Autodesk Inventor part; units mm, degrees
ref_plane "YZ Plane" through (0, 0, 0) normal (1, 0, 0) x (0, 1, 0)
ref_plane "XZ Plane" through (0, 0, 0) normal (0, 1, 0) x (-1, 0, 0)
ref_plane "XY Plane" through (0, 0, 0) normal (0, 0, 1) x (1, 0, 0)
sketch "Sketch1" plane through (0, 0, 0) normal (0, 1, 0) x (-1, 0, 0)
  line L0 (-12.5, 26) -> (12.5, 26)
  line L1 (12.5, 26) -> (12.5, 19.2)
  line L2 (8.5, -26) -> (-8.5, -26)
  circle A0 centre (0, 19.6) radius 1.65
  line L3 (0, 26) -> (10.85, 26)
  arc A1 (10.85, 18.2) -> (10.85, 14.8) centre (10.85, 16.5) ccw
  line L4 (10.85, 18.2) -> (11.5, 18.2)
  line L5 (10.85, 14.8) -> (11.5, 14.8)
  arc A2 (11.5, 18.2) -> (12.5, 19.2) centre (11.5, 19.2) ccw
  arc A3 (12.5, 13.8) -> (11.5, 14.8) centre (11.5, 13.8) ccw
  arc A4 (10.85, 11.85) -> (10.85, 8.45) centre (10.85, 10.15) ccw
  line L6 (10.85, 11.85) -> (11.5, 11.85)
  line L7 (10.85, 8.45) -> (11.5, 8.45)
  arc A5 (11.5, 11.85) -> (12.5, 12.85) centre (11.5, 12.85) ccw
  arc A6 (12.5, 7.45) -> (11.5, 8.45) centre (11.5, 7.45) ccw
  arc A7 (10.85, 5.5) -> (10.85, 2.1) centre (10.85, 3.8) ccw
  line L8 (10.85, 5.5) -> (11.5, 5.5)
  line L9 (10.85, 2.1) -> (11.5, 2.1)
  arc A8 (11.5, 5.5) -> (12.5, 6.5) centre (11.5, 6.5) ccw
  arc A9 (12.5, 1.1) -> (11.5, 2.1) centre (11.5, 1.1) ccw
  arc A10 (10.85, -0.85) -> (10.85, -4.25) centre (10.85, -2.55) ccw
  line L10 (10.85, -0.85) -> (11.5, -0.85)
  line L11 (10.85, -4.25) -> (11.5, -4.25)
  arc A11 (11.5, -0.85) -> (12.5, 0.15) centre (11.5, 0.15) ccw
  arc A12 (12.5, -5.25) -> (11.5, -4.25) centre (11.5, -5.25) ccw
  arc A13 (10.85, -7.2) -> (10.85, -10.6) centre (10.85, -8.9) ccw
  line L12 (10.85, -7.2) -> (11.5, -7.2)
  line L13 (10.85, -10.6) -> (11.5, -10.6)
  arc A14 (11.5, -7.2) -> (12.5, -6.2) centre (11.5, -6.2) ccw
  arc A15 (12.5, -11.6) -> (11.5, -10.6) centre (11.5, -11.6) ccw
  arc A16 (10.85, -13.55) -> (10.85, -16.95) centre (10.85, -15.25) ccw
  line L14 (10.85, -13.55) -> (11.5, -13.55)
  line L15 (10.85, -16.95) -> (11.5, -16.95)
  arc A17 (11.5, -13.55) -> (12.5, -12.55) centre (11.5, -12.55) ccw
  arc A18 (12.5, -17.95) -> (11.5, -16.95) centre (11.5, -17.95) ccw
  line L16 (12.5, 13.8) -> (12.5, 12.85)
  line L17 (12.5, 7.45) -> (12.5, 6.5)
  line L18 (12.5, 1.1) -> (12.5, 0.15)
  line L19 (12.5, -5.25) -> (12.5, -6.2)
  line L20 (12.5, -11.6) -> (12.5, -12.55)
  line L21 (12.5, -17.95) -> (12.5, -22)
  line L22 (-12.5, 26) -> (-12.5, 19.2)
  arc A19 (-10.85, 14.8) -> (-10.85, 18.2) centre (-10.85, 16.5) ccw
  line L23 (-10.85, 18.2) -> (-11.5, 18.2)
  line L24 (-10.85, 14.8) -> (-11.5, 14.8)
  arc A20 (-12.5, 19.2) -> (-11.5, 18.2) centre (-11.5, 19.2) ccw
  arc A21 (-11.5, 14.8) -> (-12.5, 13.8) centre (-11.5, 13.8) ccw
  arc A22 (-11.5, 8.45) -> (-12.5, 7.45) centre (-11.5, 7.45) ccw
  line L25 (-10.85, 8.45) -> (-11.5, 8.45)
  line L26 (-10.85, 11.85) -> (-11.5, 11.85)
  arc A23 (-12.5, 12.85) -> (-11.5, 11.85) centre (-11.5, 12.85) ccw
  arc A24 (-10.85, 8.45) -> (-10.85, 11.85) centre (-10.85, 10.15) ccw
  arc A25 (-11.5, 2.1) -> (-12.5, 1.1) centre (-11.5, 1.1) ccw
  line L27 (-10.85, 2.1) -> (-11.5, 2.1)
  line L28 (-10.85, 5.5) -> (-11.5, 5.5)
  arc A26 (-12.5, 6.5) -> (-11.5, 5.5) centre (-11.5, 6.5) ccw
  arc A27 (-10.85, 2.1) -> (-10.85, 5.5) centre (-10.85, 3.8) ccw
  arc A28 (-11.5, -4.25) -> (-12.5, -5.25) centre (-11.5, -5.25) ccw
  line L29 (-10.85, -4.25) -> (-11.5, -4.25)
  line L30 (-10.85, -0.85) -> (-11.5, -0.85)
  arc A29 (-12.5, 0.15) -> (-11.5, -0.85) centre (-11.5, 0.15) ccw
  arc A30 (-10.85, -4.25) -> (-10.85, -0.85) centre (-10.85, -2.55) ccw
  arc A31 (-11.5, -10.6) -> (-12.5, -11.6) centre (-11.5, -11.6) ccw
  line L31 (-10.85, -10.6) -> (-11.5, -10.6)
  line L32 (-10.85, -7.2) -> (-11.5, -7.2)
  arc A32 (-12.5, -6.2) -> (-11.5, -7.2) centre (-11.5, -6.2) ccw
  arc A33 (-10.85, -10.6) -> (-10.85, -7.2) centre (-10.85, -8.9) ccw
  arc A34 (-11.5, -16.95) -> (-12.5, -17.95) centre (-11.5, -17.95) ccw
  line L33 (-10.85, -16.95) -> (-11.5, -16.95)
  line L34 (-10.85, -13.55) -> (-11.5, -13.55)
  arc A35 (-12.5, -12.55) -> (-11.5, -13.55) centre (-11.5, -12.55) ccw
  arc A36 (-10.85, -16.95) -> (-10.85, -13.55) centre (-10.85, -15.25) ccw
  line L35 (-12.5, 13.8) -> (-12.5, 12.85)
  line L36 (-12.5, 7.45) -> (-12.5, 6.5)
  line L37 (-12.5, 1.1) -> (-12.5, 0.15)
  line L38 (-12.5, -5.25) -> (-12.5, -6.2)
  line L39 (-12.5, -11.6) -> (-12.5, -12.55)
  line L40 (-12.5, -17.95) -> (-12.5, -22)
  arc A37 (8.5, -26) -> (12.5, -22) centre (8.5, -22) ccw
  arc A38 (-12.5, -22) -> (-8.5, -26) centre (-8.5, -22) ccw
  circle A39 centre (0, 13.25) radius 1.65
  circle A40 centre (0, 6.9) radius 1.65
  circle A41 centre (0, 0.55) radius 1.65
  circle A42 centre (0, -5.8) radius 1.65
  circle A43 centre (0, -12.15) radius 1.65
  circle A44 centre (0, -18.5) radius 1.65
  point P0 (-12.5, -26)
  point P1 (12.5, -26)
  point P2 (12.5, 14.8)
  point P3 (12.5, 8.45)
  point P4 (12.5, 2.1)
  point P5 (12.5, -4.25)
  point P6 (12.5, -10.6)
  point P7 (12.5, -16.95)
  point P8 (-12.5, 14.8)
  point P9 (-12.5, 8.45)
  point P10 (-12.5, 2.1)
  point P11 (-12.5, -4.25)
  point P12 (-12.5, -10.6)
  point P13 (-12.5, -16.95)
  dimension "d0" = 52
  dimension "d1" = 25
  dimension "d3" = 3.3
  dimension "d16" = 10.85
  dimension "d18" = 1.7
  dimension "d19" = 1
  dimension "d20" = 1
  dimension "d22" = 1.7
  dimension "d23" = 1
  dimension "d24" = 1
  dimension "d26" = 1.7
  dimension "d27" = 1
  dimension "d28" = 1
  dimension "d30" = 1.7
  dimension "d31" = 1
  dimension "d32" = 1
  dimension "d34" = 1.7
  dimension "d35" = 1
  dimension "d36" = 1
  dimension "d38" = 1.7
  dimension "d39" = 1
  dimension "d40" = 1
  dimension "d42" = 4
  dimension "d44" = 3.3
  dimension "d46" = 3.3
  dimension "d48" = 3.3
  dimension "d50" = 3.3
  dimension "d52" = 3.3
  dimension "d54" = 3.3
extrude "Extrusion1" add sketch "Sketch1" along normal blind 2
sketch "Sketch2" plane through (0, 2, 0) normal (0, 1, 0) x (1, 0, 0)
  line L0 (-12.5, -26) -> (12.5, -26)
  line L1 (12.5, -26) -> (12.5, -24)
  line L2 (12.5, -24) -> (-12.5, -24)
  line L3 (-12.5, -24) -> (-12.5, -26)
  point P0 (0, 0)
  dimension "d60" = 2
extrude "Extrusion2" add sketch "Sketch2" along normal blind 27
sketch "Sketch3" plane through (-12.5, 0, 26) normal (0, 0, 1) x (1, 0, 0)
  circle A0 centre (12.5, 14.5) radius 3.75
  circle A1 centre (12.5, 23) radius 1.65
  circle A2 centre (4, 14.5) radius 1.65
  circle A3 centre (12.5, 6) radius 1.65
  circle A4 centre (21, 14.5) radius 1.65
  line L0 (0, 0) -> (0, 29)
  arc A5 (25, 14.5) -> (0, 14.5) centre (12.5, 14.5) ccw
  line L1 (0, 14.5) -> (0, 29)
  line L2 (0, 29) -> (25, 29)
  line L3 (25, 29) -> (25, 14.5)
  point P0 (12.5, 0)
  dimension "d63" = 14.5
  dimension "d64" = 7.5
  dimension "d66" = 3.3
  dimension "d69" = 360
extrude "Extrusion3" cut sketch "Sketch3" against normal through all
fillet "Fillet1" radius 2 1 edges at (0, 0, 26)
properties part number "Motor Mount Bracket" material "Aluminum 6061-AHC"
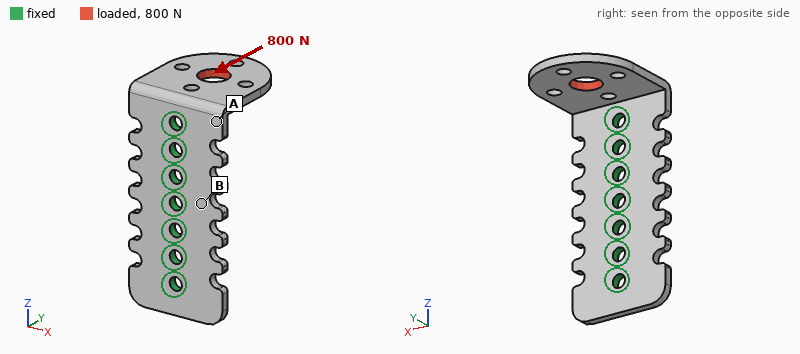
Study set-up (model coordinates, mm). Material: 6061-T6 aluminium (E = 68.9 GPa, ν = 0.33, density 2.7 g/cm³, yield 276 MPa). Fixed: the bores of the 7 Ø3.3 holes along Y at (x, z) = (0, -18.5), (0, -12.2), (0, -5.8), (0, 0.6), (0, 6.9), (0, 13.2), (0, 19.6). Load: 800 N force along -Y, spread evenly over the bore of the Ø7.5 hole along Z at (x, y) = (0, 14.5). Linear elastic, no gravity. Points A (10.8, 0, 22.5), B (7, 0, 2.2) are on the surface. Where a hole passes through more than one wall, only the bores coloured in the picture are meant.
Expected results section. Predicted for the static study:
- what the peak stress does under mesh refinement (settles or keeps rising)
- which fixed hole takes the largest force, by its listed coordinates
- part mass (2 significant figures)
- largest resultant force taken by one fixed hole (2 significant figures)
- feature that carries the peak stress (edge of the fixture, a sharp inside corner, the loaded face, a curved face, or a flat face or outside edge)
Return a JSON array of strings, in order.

["keeps rising", "(0, 19.6)", "8.5 g", "950 N", "edge of the fixture"]
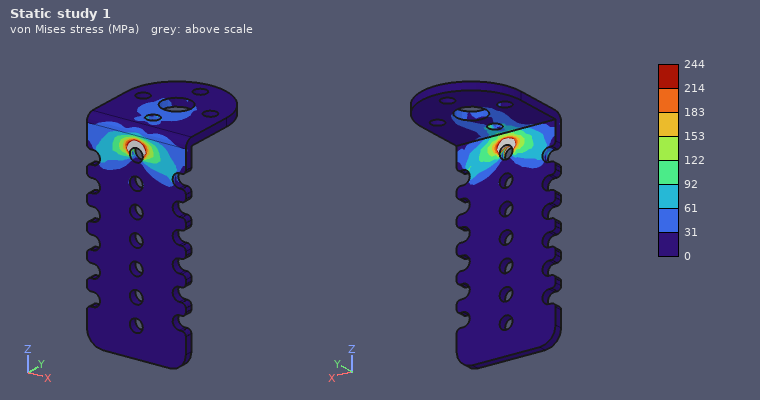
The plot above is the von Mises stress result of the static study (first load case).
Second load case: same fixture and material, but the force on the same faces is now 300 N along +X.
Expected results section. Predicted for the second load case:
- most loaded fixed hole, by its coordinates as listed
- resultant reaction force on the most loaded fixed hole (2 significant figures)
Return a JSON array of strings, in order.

["(0, 19.6)", "350 N"]
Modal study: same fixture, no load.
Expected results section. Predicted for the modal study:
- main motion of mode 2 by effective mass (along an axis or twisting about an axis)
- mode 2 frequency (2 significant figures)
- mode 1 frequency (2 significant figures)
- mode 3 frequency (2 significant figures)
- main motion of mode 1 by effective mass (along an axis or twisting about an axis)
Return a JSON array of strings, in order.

["along X", "3600 Hz", "2200 Hz", "6700 Hz", "along Z"]
